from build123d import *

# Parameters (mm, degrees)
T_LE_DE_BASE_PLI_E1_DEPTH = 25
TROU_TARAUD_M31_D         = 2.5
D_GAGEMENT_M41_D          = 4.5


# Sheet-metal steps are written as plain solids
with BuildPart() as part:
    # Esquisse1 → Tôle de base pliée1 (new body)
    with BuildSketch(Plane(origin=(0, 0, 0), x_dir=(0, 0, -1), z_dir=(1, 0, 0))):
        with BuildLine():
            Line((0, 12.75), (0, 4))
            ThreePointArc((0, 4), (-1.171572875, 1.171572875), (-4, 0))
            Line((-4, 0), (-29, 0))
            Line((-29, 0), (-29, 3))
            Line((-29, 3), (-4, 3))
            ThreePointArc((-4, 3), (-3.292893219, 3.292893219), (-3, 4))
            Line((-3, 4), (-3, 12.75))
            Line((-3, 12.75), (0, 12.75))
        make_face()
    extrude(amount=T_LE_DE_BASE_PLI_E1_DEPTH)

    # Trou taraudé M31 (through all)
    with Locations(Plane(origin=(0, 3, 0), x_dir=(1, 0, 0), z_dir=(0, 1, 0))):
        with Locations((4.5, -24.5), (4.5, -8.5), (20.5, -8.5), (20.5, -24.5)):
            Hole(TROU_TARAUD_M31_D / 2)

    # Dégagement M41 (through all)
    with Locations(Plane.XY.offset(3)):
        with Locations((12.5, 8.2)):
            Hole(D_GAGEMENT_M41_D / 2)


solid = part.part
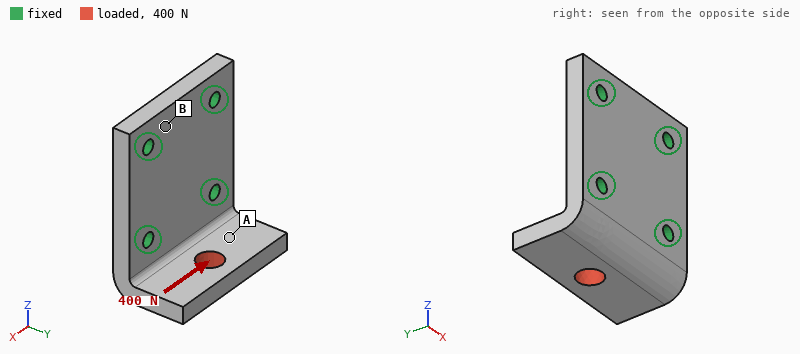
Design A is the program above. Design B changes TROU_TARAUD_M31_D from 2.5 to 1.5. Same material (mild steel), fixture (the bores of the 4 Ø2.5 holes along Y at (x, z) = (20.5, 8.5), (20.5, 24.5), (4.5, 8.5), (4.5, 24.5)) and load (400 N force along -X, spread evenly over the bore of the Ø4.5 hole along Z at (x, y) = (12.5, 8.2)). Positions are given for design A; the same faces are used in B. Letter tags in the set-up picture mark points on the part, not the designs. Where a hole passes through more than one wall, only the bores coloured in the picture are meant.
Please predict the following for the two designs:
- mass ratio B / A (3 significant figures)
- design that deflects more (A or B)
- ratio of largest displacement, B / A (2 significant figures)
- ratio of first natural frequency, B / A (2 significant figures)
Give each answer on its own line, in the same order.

1.01
B
1.2
0.92
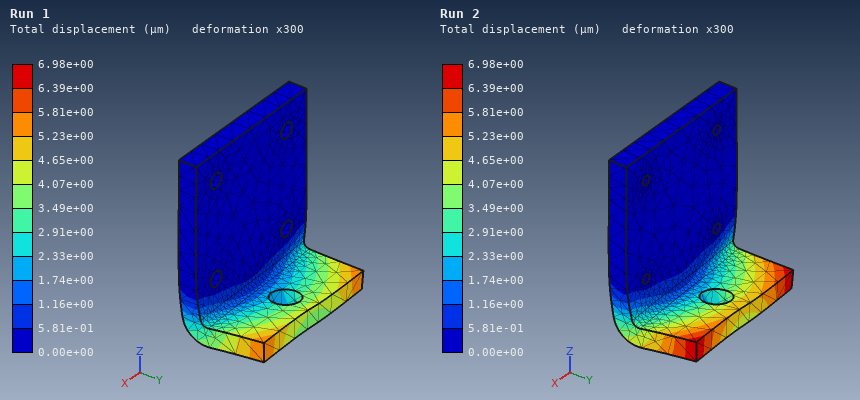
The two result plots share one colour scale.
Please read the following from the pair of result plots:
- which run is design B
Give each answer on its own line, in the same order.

Run 2
